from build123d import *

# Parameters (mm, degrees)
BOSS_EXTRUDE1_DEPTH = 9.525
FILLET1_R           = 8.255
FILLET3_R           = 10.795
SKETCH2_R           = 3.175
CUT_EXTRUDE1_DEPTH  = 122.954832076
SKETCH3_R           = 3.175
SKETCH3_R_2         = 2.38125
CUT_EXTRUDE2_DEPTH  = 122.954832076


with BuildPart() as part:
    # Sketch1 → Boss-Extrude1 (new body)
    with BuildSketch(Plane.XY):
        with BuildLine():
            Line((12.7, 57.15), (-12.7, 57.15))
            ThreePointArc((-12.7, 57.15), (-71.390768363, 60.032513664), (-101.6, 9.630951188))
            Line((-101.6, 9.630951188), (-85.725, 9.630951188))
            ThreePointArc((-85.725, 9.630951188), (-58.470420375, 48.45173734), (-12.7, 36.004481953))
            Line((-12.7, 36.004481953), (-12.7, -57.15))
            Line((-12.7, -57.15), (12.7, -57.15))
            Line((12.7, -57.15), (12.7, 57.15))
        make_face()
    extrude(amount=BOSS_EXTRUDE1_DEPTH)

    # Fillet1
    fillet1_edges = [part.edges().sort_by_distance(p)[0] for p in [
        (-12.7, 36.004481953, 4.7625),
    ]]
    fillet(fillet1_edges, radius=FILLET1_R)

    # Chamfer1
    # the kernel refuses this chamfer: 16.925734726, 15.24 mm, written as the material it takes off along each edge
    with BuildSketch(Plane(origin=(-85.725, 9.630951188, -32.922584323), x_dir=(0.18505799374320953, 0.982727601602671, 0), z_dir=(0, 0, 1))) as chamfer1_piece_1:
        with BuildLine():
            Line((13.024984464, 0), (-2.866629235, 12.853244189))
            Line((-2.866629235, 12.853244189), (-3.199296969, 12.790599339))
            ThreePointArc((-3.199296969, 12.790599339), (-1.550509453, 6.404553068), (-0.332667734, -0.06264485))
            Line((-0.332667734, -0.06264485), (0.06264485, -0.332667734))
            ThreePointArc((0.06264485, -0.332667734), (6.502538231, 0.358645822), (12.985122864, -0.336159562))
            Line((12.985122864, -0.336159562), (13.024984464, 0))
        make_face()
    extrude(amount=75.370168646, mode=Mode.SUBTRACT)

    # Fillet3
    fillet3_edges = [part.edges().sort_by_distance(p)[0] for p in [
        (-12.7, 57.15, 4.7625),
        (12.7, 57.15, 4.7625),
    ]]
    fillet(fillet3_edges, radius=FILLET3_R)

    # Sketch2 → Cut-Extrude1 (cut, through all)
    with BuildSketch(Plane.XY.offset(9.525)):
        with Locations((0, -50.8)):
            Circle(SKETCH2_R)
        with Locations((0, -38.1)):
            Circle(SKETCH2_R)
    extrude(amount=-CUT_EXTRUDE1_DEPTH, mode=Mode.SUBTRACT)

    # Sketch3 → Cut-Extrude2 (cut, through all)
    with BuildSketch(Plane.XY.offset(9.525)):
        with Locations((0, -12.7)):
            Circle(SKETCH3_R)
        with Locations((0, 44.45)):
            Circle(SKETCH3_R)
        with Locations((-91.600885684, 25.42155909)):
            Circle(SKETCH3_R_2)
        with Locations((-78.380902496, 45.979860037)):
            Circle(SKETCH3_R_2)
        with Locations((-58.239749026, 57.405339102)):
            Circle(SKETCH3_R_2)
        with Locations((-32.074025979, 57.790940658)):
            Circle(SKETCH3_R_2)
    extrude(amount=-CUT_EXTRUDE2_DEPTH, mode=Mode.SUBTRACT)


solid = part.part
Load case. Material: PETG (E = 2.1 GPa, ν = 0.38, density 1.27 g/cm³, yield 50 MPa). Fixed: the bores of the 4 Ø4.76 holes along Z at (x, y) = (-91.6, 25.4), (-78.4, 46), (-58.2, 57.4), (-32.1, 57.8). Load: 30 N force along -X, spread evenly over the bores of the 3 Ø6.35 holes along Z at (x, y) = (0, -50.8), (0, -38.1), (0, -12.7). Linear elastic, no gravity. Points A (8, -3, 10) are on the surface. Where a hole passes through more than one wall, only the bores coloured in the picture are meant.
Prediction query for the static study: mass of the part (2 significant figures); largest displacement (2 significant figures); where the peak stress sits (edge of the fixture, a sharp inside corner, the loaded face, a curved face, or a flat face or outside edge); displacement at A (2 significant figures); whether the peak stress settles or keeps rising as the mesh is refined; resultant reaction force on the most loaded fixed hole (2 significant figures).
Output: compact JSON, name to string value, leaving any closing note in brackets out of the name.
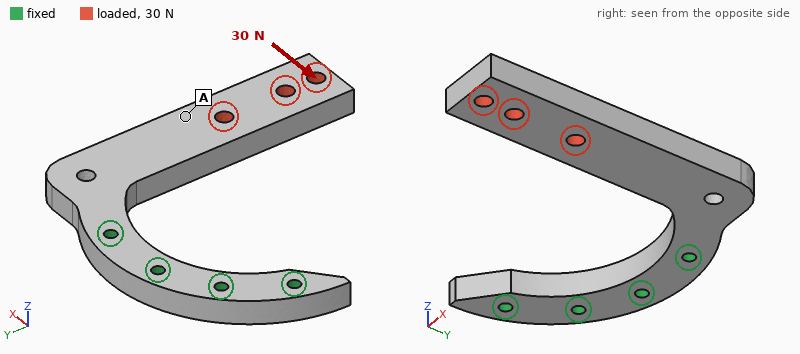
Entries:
{"mass of the part": "53 g", "largest displacement": "1.7 mm", "where the peak stress sits": "edge of the fixture", "displacement at A": "0.86 mm", "whether the peak stress settles or keeps rising as the mesh is refined": "keeps rising", "resultant reaction force on the most loaded fixed hole": "62 N"}
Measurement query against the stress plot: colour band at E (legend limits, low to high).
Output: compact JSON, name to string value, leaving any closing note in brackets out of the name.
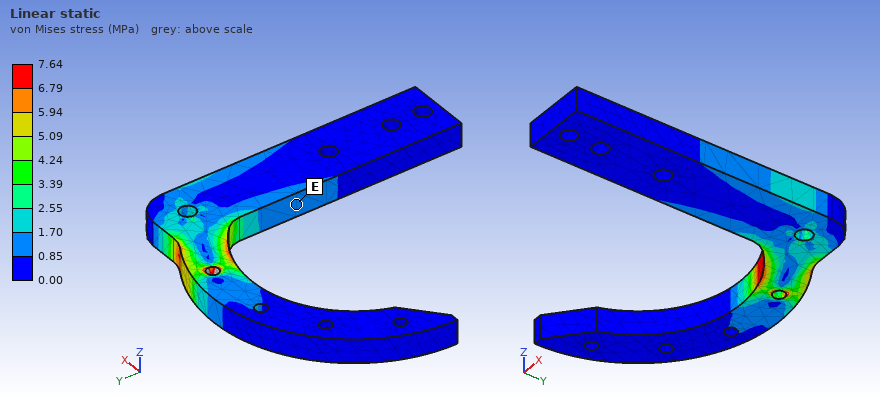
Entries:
{"colour band at E": "0.85 to 1.70 MPa"}
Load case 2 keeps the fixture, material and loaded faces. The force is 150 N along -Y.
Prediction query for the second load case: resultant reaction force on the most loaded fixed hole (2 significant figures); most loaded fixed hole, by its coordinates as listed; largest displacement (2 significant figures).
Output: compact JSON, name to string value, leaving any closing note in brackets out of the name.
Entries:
{"resultant reaction force on the most loaded fixed hole": "250 N", "most loaded fixed hole, by its coordinates as listed": "(-32.1, 57.8)", "largest displacement": "1.9 mm"}
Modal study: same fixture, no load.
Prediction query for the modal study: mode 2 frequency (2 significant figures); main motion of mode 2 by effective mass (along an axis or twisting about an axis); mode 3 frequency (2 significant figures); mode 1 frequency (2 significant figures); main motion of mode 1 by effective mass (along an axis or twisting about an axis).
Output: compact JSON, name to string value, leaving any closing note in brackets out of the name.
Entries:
{"mode 2 frequency": "180 Hz", "main motion of mode 2 by effective mass": "along X", "mode 3 frequency": "510 Hz", "mode 1 frequency": "110 Hz", "main motion of mode 1 by effective mass": "along Z"}
